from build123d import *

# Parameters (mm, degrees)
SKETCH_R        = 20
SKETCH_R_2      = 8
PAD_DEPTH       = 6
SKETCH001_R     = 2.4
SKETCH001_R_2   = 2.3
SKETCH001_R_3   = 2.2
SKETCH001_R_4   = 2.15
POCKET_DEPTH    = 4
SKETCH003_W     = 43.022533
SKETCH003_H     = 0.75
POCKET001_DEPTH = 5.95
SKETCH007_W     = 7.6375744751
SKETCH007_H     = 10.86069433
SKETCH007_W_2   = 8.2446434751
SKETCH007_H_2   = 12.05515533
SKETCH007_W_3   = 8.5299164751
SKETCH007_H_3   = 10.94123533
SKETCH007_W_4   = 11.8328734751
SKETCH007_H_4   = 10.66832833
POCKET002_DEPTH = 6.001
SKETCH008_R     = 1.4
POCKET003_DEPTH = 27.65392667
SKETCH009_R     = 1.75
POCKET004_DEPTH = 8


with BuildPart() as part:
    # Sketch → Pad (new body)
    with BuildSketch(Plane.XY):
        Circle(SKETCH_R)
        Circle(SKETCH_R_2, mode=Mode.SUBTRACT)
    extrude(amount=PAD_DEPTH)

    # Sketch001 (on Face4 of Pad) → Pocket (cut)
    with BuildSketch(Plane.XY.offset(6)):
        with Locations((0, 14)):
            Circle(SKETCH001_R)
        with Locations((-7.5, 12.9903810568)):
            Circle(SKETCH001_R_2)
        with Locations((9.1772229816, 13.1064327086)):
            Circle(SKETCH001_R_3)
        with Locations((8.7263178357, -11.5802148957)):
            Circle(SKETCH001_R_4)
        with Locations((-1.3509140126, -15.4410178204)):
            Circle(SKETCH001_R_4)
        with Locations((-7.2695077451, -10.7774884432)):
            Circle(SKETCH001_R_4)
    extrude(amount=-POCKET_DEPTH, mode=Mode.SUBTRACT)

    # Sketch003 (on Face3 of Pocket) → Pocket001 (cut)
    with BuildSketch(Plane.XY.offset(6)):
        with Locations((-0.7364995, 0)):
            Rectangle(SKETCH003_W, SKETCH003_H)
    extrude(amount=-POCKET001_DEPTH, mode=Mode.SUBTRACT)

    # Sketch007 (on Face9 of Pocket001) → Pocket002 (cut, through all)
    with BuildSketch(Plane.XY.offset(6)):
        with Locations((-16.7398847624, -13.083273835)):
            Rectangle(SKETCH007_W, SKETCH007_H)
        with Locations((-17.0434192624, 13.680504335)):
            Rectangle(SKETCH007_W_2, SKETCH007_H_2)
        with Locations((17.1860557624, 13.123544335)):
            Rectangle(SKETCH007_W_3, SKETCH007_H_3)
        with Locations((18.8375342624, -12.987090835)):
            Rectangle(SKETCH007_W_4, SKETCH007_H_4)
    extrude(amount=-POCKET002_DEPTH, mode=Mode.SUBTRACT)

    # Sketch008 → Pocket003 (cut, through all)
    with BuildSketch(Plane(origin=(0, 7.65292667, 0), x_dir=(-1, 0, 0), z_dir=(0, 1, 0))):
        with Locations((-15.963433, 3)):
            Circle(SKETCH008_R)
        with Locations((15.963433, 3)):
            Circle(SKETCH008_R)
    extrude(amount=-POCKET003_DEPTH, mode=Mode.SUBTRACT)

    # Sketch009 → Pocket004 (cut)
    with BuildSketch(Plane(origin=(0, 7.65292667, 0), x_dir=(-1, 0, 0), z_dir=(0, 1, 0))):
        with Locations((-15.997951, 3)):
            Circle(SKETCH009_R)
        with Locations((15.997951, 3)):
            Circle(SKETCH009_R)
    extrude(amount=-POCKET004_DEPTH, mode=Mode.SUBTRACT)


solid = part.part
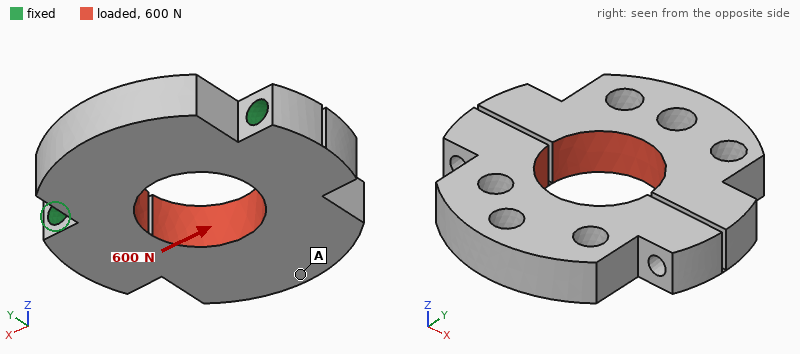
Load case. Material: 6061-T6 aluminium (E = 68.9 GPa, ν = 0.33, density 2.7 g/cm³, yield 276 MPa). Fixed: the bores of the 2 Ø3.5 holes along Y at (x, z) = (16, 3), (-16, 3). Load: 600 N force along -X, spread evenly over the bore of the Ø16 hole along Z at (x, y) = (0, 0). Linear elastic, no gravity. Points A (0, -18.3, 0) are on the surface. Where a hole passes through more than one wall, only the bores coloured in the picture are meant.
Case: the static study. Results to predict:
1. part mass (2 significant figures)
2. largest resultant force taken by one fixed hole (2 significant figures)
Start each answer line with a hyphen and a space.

- 14 g
- 310 N
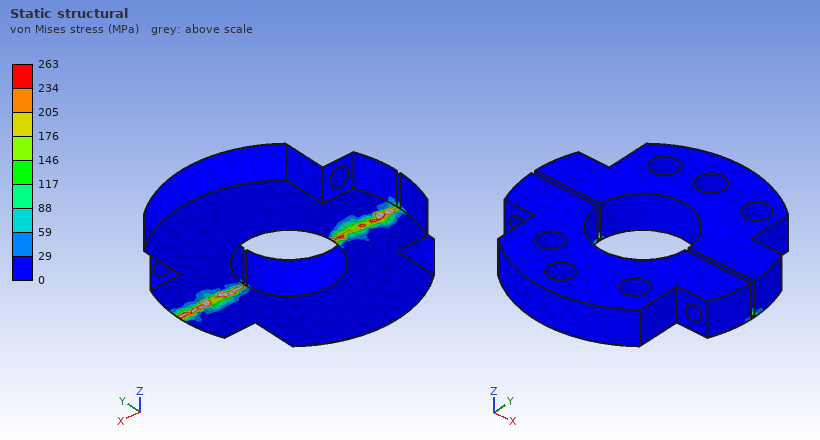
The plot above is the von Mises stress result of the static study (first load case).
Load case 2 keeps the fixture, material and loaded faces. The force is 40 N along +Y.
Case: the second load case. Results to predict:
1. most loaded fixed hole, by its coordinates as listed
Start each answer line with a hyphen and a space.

- (-16, 3)
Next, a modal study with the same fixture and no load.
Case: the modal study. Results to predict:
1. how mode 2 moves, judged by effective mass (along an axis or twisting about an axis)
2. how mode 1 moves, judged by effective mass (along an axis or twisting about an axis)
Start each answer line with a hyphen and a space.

- along X
- along Z
